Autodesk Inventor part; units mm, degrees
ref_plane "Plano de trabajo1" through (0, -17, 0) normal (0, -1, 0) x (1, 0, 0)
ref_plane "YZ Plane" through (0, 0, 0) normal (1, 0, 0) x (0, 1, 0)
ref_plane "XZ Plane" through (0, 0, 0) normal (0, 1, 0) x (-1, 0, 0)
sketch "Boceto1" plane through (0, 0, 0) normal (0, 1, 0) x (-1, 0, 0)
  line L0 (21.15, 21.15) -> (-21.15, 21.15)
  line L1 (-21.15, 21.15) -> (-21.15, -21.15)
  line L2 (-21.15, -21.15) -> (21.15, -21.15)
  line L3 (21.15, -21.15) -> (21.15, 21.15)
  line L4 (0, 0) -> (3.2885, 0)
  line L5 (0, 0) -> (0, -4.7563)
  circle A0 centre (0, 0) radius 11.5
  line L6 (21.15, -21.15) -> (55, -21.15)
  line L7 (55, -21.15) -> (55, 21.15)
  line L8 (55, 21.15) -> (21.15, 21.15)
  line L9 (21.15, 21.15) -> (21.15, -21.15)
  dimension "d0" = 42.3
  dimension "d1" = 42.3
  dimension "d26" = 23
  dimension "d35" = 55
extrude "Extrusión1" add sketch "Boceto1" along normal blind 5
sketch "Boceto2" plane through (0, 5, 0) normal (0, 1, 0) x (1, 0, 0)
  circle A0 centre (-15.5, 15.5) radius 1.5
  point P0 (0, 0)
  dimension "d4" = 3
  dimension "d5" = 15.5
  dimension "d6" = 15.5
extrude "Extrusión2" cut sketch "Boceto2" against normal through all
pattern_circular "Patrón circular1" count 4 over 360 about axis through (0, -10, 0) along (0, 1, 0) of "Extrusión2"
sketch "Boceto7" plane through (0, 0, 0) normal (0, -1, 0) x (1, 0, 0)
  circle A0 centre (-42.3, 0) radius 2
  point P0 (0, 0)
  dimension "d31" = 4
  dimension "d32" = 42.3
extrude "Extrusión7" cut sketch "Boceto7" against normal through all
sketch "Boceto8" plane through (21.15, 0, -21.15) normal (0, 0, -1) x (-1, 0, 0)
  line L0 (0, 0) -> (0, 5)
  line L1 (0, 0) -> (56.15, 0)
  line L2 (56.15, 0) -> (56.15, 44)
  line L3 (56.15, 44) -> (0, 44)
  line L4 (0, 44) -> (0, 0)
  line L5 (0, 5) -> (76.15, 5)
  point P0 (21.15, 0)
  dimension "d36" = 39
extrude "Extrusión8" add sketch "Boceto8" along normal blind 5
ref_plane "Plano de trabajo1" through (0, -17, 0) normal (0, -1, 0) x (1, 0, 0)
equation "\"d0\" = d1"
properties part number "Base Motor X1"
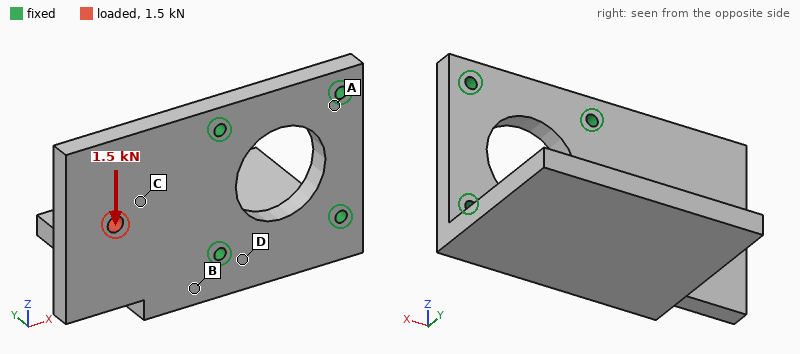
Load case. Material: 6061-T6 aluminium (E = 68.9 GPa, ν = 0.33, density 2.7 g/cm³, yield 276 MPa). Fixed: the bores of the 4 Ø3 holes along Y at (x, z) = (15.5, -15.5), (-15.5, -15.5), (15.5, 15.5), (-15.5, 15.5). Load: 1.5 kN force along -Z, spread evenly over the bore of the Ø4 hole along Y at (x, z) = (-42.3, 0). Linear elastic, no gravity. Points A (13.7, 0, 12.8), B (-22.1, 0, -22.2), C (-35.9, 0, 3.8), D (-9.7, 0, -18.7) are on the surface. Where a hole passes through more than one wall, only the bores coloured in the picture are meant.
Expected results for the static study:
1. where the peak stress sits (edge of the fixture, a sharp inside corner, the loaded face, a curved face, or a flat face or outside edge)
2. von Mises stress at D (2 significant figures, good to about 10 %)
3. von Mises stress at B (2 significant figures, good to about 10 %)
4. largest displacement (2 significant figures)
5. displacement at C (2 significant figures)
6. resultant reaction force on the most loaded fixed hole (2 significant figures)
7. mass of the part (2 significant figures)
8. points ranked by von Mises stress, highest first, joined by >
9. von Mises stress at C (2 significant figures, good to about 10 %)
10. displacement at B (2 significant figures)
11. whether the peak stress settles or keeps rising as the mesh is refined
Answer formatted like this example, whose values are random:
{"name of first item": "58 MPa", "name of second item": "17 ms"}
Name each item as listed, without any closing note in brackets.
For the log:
{"where the peak stress sits": "edge of the fixture", "von Mises stress at D": "7.4 MPa", "von Mises stress at B": "11 MPa", "largest displacement": "17 µm", "displacement at C": "9.4 µm", "resultant reaction force on the most loaded fixed hole": "1.3 kN", "mass of the part": "71 g", "points ranked by von Mises stress, highest first, joined by >": "C > B > D > A", "von Mises stress at C": "16 MPa", "displacement at B": "4.6 µm", "whether the peak stress settles or keeps rising as the mesh is refined": "keeps rising"}
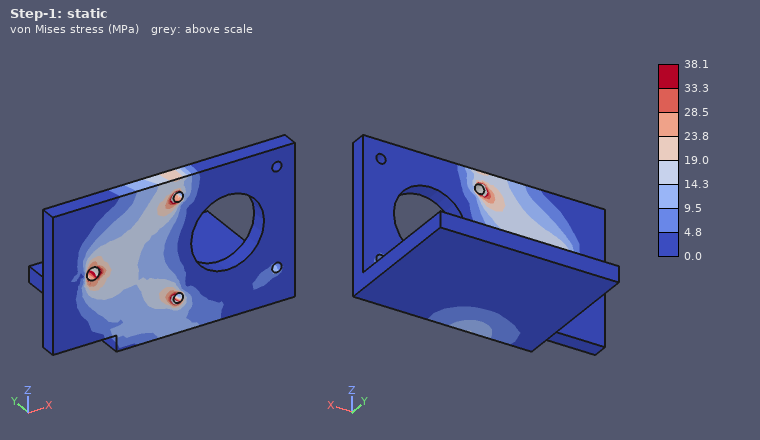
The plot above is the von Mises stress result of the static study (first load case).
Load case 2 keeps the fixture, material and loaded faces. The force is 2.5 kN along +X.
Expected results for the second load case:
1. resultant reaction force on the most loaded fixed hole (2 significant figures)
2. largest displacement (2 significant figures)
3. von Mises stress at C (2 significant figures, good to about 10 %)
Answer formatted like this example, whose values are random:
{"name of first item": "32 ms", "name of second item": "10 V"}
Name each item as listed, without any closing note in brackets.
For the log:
{"resultant reaction force on the most loaded fixed hole": "1.2 kN", "largest displacement": "11 µm", "von Mises stress at C": "24 MPa"}
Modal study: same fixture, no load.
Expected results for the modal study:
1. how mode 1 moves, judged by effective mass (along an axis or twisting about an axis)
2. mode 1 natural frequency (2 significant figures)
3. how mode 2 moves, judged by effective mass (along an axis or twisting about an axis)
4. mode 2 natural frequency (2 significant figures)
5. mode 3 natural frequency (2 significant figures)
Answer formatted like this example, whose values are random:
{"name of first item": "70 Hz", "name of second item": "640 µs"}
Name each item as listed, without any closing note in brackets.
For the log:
{"how mode 1 moves, judged by effective mass": "along Z", "mode 1 natural frequency": "1700 Hz", "how mode 2 moves, judged by effective mass": "along Y", "mode 2 natural frequency": "3000 Hz", "mode 3 natural frequency": "3900 Hz"}
